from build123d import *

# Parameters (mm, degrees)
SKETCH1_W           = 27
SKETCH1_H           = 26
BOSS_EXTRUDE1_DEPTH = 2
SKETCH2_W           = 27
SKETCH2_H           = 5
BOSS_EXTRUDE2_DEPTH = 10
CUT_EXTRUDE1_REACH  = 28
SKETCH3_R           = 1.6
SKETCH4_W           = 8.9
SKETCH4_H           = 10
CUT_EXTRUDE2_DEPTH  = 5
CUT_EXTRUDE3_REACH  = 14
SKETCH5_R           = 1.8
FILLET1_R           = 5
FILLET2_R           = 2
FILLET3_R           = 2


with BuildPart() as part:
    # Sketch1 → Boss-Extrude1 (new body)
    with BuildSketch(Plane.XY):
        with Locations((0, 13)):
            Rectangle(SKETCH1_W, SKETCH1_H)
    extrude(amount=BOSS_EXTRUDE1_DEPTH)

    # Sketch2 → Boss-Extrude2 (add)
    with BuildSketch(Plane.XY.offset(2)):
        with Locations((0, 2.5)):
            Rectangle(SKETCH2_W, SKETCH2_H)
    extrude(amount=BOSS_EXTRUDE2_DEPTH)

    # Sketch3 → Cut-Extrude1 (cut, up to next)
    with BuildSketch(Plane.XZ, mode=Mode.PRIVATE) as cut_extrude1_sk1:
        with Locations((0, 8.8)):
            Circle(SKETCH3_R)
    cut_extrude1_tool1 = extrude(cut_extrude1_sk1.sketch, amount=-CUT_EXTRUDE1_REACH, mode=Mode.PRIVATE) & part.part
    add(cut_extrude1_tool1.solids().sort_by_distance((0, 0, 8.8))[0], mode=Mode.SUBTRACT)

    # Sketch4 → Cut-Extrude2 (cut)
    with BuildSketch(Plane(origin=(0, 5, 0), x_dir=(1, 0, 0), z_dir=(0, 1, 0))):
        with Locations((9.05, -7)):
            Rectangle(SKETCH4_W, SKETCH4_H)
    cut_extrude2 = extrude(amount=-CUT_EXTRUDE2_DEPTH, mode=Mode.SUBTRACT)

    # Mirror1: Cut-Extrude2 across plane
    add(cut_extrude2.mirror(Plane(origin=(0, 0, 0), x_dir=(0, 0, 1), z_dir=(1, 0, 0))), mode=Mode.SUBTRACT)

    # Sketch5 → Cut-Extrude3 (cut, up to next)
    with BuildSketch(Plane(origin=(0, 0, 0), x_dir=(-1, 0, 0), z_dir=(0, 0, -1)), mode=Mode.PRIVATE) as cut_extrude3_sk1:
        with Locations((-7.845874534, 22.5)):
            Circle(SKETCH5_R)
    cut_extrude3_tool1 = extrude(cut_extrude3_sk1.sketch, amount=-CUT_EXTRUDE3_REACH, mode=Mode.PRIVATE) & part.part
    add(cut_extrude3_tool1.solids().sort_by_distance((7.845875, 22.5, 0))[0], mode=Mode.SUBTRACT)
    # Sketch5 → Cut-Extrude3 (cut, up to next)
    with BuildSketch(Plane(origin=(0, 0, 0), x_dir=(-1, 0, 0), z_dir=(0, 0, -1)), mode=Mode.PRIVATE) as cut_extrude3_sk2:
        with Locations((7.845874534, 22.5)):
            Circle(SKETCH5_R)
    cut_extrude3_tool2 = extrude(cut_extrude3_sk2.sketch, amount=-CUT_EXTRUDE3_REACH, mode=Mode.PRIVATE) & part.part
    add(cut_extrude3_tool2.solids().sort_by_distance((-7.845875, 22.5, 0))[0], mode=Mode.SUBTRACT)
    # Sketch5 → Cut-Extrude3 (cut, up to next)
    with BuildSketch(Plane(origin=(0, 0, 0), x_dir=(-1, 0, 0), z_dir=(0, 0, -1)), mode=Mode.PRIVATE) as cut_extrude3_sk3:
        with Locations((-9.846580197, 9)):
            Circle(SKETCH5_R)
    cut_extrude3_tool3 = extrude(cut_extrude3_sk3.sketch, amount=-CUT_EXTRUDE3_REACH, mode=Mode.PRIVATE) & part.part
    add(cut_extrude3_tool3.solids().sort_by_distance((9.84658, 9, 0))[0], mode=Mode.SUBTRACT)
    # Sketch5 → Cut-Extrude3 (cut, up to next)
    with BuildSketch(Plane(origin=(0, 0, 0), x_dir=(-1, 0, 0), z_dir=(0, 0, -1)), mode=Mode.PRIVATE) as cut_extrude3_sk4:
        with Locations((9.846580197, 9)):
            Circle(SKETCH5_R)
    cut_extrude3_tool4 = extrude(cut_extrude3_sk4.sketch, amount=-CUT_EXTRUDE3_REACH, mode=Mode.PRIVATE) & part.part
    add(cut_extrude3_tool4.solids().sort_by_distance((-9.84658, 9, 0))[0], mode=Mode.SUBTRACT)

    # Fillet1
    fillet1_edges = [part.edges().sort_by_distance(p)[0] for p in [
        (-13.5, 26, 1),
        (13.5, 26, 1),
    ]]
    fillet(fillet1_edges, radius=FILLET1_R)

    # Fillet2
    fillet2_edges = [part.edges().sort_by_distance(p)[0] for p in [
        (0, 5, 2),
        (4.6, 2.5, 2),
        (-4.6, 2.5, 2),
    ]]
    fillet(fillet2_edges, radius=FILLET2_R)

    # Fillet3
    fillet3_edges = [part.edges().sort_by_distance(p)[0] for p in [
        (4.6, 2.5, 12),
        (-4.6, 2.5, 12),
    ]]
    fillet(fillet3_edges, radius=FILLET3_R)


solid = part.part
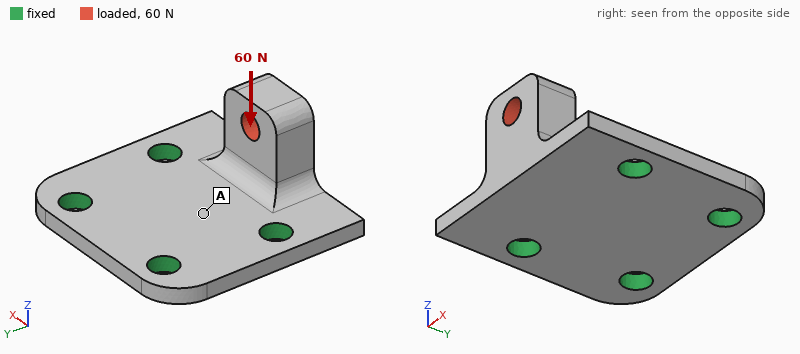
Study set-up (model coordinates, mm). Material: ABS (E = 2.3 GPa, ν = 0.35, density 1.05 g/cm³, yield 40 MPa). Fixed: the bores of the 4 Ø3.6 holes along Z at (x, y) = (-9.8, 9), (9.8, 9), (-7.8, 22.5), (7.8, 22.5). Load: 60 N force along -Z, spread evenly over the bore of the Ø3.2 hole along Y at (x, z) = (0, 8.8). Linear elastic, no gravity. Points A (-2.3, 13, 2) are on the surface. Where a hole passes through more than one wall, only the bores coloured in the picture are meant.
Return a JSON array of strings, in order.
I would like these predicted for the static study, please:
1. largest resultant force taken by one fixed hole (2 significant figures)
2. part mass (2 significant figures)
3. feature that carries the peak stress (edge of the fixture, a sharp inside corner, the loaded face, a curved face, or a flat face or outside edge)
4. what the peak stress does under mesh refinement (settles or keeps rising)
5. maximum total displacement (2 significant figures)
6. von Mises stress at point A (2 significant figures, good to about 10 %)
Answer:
["34 N", "1.8 g", "edge of the fixture", "keeps rising", "0.39 mm", "3.9 MPa"]
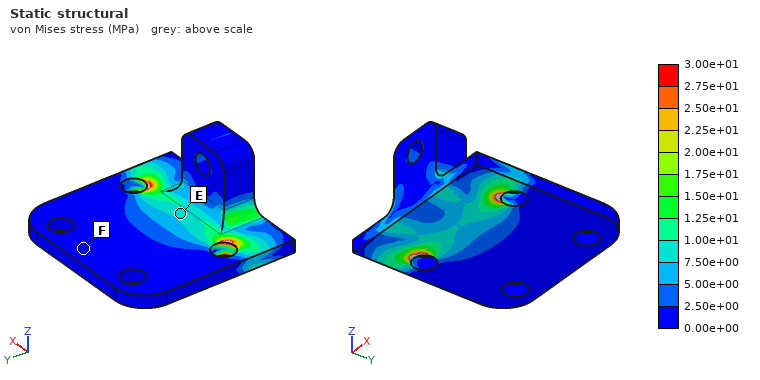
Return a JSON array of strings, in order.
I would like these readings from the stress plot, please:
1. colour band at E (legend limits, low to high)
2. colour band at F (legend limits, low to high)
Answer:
["7.50e+00 to 1.00e+01 MPa", "0.00e+00 to 2.50e+00 MPa"]
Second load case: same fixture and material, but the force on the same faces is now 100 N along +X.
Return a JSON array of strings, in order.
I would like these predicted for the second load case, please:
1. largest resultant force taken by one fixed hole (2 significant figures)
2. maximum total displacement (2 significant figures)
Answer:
["76 N", "0.26 mm"]
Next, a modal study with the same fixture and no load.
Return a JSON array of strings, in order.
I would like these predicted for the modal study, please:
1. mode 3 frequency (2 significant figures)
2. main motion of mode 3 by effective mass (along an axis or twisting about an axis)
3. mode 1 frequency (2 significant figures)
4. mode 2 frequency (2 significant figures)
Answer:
["6900 Hz", "along Z", "2600 Hz", "6100 Hz"]
